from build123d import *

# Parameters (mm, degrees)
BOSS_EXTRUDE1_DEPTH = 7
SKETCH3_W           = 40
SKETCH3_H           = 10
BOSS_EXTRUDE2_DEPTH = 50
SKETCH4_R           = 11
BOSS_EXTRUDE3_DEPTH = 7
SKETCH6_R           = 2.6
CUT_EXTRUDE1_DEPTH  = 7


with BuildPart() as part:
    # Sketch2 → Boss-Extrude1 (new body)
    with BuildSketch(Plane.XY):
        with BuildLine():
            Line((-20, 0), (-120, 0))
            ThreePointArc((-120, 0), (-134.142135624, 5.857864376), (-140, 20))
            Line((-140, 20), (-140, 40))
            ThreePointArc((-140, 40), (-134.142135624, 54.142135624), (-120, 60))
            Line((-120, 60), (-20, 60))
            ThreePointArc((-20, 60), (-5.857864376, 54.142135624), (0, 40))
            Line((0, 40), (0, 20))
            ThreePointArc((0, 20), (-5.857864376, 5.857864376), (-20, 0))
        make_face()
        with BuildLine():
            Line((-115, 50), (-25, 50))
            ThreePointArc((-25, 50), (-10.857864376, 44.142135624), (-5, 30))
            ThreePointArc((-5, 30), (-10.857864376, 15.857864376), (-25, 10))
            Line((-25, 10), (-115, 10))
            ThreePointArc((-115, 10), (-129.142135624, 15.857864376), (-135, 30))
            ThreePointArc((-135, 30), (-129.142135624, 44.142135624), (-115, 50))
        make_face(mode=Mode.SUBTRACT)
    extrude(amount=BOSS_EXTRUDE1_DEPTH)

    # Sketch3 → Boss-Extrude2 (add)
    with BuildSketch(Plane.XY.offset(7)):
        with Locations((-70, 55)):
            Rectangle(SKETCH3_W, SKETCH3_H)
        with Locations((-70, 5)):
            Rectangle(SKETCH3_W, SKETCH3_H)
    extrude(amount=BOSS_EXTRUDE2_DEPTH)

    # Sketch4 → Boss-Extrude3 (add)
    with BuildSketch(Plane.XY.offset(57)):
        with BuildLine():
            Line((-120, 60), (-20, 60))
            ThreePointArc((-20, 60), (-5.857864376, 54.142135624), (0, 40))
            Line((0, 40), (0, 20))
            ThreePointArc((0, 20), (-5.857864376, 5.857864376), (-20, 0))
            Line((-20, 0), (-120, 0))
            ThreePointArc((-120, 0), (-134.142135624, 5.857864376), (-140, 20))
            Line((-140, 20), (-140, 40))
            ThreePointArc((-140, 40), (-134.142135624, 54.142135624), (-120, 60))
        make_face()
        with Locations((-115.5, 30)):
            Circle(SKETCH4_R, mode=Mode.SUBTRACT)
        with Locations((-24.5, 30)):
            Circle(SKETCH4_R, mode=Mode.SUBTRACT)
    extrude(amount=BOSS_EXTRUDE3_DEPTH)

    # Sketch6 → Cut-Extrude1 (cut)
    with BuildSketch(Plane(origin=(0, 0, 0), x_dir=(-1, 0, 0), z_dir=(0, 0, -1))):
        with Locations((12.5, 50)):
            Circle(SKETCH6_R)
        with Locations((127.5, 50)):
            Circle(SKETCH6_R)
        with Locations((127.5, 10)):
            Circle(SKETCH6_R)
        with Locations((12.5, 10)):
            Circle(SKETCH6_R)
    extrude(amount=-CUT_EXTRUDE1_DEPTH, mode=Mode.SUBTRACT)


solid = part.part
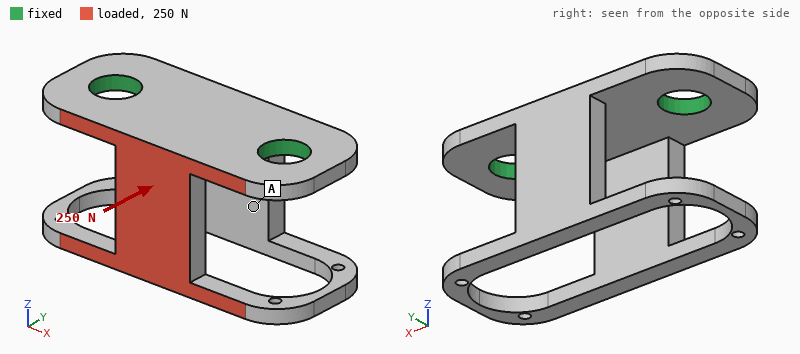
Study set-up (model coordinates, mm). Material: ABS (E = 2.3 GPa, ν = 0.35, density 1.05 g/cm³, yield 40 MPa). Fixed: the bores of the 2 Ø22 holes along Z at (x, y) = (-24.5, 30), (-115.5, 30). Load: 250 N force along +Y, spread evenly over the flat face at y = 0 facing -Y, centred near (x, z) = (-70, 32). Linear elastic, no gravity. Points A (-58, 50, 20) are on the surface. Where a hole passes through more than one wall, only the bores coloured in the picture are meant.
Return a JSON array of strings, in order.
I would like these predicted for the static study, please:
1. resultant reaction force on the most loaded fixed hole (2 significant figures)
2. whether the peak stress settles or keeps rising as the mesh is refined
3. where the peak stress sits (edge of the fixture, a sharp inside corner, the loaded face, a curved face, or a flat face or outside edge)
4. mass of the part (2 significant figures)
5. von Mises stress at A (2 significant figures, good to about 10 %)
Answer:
["130 N", "keeps rising", "a sharp inside corner", "120 g", "1.1 MPa"]
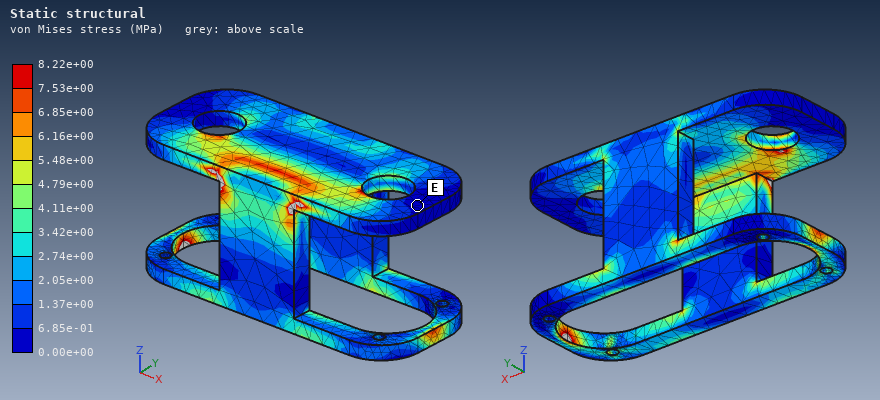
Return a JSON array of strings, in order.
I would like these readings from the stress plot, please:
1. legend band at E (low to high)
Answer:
["0.00e+00 to 6.85e-01 MPa"]
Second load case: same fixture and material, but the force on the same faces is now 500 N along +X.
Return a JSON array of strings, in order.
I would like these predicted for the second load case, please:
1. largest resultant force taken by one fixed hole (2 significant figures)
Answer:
["370 N"]
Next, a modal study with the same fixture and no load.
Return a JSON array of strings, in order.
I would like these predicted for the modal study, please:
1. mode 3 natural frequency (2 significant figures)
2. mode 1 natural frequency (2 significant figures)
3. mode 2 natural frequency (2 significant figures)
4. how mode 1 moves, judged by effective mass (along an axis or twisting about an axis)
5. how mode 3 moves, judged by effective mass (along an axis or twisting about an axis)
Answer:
["450 Hz", "260 Hz", "400 Hz", "along Y", "along Z"]
